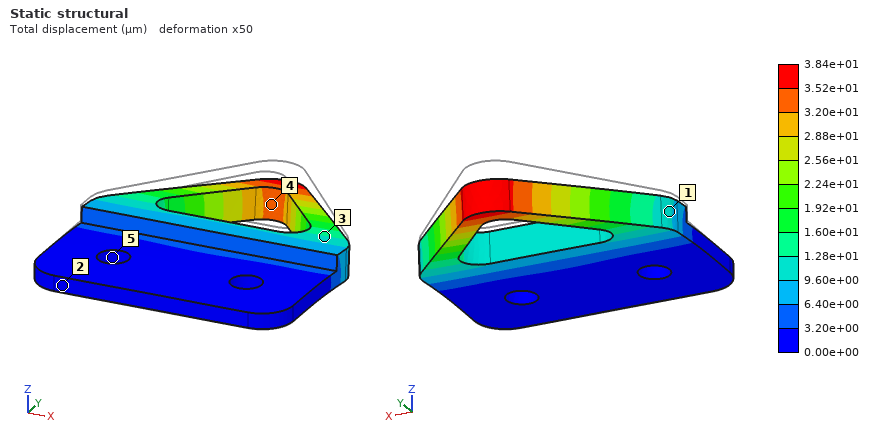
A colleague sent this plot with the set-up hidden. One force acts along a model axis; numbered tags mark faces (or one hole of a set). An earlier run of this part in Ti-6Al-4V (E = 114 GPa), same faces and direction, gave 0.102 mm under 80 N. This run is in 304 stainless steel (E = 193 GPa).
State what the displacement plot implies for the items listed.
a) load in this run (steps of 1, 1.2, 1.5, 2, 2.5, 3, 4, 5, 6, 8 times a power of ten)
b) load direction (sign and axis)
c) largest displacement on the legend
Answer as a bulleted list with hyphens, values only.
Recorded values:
- 50 N
- -Z
- 3.84e+01 µm
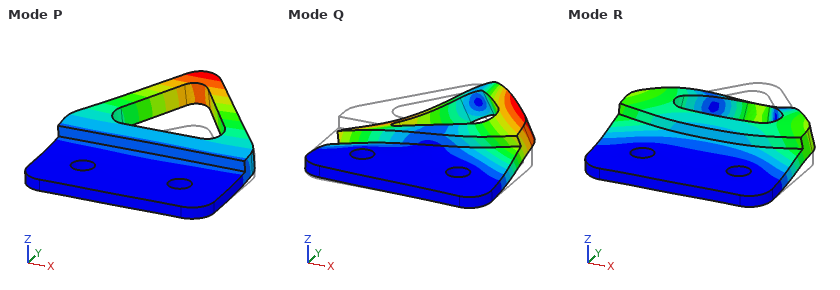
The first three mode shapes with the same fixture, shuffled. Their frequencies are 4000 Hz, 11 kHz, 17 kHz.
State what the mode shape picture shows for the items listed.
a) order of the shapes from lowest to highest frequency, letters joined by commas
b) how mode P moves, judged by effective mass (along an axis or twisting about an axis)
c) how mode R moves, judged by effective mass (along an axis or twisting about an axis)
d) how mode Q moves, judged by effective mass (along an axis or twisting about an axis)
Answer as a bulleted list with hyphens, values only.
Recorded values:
- P, Q, R
- along Z
- along Z
- twisting about Y
